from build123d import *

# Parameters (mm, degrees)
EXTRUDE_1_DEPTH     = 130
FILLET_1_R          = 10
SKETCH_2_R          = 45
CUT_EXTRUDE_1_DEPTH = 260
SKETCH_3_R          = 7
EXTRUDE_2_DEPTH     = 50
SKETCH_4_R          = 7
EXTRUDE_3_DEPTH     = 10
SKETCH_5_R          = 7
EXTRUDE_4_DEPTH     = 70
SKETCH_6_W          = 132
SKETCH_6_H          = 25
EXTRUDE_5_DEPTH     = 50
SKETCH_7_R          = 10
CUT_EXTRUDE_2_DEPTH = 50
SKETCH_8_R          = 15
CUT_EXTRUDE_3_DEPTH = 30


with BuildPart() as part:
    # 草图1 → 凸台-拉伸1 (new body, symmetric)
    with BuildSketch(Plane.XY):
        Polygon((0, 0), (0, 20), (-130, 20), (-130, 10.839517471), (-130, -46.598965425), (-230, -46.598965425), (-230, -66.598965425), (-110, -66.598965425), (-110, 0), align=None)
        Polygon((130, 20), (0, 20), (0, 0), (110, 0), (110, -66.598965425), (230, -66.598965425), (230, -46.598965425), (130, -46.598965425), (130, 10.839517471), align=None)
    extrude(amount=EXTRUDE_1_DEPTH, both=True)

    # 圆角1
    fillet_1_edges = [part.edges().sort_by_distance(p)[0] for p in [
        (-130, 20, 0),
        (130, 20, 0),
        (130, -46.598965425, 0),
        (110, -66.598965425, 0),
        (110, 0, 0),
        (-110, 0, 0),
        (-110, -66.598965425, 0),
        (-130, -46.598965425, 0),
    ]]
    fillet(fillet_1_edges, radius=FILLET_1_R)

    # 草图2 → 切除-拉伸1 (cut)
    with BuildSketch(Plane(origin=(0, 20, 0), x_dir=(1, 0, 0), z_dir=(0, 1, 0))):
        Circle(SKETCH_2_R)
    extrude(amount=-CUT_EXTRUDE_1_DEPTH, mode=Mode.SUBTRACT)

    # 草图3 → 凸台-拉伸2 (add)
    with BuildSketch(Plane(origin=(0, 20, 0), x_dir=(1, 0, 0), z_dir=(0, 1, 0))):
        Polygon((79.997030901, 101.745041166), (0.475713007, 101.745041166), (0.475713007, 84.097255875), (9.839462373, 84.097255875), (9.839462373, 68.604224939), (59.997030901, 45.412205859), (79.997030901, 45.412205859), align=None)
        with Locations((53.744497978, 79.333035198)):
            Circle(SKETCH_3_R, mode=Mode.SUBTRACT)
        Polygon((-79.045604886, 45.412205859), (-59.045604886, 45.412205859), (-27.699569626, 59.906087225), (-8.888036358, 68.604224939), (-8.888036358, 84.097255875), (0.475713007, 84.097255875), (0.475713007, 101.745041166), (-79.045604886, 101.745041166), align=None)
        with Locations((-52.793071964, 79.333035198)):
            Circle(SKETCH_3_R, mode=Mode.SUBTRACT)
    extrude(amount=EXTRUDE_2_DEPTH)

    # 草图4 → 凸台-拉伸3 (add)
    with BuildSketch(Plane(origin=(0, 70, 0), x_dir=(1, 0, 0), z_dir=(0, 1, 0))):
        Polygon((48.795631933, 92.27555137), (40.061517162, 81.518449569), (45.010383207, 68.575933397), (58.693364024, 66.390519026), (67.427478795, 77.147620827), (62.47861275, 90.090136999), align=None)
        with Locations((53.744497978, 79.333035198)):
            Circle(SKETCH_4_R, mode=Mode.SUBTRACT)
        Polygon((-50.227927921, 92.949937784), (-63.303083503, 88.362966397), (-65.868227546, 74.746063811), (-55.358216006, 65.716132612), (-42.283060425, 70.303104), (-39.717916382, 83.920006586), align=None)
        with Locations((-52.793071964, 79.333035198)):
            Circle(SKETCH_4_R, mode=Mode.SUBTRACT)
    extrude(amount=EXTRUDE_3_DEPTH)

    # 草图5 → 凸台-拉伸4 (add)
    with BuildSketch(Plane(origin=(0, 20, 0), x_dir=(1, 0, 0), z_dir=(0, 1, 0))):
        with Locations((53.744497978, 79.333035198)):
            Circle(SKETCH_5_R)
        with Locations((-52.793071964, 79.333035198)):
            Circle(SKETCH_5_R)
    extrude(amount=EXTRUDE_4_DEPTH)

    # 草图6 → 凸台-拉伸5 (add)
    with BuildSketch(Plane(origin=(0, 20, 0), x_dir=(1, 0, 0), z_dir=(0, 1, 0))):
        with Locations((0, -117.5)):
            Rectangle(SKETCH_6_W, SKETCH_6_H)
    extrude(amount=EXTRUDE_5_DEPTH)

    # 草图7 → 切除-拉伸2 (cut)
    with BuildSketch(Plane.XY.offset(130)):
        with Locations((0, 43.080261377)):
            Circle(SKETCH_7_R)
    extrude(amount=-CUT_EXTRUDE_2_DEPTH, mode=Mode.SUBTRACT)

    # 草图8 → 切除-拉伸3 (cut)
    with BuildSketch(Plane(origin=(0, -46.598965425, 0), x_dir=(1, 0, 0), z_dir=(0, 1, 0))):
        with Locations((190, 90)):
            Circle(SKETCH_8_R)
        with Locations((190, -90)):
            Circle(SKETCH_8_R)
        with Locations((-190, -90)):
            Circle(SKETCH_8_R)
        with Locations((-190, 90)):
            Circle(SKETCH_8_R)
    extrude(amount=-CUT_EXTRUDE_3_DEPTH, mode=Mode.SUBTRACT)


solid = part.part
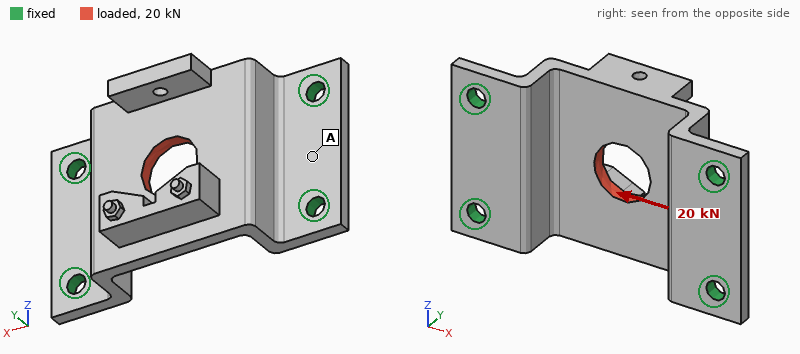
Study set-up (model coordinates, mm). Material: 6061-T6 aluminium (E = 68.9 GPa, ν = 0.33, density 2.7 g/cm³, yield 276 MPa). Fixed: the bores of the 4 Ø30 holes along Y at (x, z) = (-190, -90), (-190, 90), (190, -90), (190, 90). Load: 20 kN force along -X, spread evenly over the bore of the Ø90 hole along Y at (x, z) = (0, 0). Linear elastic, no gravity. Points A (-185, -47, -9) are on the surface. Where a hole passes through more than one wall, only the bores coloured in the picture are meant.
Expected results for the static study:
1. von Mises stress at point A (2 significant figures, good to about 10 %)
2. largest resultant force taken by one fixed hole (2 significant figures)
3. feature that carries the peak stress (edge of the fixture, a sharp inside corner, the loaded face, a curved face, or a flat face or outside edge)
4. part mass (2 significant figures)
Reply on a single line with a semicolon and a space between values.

4.5 MPa; 5.5 kN; a curved face; 9.2 kg
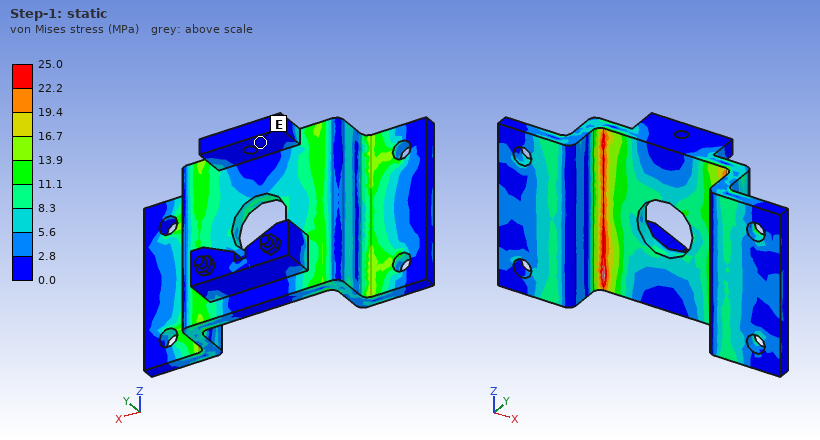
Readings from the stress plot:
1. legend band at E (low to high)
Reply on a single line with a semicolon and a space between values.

0.0 to 2.8 MPa
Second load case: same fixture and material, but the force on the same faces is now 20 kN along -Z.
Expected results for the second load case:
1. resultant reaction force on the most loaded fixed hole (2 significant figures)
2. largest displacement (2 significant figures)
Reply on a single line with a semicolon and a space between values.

7.8 kN; 61 µm
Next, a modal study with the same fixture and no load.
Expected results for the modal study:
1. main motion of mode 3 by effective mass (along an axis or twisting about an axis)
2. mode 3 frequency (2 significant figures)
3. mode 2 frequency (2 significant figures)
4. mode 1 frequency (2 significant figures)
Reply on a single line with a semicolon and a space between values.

along Y; 1300 Hz; 1200 Hz; 1100 Hz
